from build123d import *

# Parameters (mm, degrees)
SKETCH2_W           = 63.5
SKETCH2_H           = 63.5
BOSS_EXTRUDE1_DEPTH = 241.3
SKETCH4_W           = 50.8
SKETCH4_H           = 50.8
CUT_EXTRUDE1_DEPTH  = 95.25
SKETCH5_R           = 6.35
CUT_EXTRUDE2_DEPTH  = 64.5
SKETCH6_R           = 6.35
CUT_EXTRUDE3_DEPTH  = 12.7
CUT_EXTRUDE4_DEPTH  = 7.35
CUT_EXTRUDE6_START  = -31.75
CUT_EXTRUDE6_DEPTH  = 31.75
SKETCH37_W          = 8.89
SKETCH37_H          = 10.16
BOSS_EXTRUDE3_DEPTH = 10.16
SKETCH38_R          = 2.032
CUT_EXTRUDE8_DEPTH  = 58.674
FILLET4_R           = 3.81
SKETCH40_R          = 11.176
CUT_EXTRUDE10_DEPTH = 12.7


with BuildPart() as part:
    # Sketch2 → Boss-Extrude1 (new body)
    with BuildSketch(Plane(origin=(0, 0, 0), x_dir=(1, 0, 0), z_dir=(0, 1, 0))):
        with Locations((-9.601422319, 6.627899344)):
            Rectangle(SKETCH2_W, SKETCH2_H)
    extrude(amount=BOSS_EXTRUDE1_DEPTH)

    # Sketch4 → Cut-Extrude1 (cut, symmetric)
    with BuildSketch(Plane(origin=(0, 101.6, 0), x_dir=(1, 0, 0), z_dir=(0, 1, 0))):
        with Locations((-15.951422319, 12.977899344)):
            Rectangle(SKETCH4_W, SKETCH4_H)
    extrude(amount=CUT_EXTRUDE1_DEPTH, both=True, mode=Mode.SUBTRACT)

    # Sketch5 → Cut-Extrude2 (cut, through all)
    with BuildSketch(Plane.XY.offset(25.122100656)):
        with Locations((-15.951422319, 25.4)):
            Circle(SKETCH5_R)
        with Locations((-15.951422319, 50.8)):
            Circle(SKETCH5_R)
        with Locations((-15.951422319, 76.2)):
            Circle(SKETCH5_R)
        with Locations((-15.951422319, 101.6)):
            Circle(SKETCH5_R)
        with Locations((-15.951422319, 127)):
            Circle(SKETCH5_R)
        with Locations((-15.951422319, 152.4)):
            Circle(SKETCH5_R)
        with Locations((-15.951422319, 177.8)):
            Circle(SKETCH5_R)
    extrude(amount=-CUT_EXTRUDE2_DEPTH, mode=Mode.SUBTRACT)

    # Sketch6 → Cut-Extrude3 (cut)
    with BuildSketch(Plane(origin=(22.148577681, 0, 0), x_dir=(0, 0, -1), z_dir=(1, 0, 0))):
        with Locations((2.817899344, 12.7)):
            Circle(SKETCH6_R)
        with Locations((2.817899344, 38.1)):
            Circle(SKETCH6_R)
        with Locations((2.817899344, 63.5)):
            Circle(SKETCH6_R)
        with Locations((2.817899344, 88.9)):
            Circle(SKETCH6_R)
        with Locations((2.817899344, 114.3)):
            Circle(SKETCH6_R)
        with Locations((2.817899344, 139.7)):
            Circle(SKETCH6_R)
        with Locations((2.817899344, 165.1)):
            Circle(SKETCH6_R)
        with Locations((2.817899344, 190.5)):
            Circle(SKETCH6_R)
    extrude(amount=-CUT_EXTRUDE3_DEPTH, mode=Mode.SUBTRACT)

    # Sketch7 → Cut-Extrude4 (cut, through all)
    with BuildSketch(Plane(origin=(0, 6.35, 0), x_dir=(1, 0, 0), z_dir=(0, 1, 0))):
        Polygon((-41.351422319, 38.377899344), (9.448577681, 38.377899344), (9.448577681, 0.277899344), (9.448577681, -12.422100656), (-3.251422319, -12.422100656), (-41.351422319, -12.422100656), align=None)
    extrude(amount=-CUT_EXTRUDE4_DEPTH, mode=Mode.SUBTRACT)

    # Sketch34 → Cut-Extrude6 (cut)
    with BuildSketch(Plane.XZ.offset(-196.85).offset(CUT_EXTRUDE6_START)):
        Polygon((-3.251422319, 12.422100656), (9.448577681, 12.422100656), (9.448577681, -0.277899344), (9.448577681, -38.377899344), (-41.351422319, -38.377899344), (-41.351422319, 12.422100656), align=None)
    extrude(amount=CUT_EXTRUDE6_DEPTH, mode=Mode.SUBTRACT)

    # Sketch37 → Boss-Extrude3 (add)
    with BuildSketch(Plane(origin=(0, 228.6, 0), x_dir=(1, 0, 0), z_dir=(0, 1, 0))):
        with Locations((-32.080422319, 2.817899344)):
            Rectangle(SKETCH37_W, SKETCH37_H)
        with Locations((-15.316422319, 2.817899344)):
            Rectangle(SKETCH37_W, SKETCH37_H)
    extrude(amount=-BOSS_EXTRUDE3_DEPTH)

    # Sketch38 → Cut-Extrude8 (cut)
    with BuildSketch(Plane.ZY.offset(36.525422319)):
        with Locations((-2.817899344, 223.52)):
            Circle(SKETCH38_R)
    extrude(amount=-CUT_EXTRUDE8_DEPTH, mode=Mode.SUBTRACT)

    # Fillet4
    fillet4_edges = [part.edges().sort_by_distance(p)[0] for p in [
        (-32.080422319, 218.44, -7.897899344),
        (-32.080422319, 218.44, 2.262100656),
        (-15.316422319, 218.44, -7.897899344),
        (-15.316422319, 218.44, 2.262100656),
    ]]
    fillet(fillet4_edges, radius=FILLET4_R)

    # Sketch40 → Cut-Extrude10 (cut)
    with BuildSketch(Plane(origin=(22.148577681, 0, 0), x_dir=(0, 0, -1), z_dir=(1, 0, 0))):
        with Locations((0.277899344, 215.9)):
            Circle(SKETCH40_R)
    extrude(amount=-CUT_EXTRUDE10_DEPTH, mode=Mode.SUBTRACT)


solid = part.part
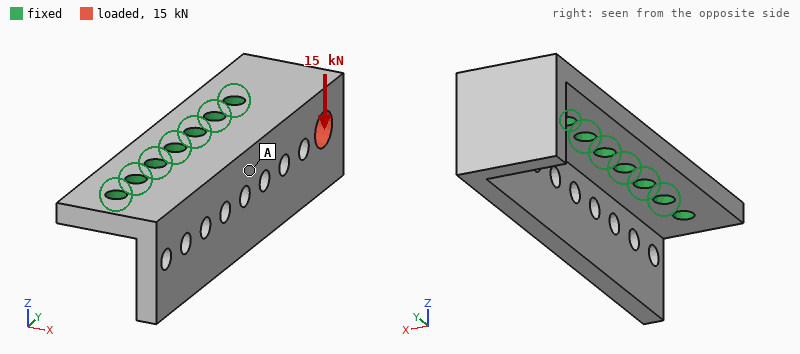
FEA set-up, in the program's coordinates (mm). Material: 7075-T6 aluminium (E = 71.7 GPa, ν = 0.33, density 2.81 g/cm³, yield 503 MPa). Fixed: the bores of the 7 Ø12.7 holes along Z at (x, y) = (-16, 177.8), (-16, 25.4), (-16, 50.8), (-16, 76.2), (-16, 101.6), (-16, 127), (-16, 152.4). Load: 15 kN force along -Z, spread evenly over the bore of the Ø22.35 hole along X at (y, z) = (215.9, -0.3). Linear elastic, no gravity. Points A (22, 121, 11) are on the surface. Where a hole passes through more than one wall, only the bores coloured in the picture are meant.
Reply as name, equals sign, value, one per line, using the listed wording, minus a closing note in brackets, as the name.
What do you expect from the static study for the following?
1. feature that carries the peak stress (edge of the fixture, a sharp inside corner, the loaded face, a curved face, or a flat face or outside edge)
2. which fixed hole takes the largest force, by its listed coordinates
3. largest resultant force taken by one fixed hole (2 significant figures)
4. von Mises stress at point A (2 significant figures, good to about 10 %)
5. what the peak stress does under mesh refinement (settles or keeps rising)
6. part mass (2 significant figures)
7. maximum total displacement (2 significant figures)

feature that carries the peak stress = edge of the fixture
which fixed hole takes the largest force, by its listed coordinates = (-16, 177.8)
largest resultant force taken by one fixed hole = 14 kN
von Mises stress at point A = 28 MPa
what the peak stress does under mesh refinement = keeps rising
part mass = 1000 g
maximum total displacement = 0.59 mm
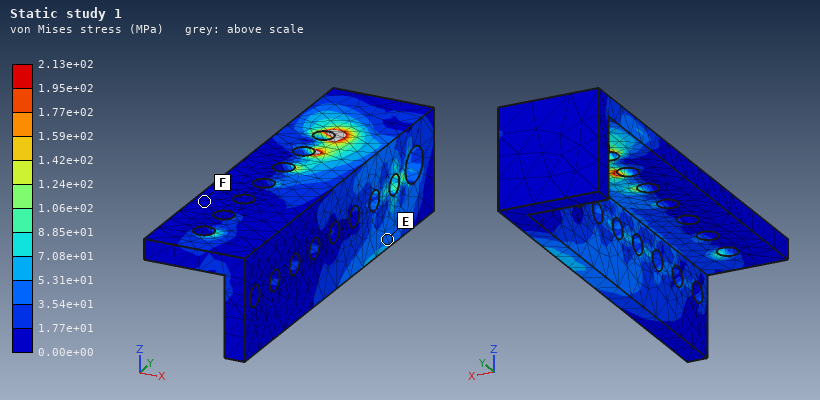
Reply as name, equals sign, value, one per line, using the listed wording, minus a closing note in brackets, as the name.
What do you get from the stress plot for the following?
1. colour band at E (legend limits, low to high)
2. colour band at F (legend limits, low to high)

colour band at E = 3.54e+01 to 5.31e+01 MPa
colour band at F = 0.00e+00 to 1.77e+01 MPa
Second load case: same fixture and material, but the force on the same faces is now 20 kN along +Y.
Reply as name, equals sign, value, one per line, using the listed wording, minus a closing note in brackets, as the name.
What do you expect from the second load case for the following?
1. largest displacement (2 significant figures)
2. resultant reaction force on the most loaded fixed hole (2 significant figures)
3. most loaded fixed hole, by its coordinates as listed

largest displacement = 91 µm
resultant reaction force on the most loaded fixed hole = 9.2 kN
most loaded fixed hole, by its coordinates as listed = (-16, 177.8)
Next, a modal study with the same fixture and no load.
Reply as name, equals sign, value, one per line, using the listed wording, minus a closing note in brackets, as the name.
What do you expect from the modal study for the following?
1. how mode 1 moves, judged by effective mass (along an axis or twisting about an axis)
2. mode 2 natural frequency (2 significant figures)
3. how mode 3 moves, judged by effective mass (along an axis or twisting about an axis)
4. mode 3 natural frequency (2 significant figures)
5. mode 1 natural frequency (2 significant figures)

how mode 1 moves, judged by effective mass = along X
mode 2 natural frequency = 2000 Hz
how mode 3 moves, judged by effective mass = along Z
mode 3 natural frequency = 2300 Hz
mode 1 natural frequency = 1600 Hz
